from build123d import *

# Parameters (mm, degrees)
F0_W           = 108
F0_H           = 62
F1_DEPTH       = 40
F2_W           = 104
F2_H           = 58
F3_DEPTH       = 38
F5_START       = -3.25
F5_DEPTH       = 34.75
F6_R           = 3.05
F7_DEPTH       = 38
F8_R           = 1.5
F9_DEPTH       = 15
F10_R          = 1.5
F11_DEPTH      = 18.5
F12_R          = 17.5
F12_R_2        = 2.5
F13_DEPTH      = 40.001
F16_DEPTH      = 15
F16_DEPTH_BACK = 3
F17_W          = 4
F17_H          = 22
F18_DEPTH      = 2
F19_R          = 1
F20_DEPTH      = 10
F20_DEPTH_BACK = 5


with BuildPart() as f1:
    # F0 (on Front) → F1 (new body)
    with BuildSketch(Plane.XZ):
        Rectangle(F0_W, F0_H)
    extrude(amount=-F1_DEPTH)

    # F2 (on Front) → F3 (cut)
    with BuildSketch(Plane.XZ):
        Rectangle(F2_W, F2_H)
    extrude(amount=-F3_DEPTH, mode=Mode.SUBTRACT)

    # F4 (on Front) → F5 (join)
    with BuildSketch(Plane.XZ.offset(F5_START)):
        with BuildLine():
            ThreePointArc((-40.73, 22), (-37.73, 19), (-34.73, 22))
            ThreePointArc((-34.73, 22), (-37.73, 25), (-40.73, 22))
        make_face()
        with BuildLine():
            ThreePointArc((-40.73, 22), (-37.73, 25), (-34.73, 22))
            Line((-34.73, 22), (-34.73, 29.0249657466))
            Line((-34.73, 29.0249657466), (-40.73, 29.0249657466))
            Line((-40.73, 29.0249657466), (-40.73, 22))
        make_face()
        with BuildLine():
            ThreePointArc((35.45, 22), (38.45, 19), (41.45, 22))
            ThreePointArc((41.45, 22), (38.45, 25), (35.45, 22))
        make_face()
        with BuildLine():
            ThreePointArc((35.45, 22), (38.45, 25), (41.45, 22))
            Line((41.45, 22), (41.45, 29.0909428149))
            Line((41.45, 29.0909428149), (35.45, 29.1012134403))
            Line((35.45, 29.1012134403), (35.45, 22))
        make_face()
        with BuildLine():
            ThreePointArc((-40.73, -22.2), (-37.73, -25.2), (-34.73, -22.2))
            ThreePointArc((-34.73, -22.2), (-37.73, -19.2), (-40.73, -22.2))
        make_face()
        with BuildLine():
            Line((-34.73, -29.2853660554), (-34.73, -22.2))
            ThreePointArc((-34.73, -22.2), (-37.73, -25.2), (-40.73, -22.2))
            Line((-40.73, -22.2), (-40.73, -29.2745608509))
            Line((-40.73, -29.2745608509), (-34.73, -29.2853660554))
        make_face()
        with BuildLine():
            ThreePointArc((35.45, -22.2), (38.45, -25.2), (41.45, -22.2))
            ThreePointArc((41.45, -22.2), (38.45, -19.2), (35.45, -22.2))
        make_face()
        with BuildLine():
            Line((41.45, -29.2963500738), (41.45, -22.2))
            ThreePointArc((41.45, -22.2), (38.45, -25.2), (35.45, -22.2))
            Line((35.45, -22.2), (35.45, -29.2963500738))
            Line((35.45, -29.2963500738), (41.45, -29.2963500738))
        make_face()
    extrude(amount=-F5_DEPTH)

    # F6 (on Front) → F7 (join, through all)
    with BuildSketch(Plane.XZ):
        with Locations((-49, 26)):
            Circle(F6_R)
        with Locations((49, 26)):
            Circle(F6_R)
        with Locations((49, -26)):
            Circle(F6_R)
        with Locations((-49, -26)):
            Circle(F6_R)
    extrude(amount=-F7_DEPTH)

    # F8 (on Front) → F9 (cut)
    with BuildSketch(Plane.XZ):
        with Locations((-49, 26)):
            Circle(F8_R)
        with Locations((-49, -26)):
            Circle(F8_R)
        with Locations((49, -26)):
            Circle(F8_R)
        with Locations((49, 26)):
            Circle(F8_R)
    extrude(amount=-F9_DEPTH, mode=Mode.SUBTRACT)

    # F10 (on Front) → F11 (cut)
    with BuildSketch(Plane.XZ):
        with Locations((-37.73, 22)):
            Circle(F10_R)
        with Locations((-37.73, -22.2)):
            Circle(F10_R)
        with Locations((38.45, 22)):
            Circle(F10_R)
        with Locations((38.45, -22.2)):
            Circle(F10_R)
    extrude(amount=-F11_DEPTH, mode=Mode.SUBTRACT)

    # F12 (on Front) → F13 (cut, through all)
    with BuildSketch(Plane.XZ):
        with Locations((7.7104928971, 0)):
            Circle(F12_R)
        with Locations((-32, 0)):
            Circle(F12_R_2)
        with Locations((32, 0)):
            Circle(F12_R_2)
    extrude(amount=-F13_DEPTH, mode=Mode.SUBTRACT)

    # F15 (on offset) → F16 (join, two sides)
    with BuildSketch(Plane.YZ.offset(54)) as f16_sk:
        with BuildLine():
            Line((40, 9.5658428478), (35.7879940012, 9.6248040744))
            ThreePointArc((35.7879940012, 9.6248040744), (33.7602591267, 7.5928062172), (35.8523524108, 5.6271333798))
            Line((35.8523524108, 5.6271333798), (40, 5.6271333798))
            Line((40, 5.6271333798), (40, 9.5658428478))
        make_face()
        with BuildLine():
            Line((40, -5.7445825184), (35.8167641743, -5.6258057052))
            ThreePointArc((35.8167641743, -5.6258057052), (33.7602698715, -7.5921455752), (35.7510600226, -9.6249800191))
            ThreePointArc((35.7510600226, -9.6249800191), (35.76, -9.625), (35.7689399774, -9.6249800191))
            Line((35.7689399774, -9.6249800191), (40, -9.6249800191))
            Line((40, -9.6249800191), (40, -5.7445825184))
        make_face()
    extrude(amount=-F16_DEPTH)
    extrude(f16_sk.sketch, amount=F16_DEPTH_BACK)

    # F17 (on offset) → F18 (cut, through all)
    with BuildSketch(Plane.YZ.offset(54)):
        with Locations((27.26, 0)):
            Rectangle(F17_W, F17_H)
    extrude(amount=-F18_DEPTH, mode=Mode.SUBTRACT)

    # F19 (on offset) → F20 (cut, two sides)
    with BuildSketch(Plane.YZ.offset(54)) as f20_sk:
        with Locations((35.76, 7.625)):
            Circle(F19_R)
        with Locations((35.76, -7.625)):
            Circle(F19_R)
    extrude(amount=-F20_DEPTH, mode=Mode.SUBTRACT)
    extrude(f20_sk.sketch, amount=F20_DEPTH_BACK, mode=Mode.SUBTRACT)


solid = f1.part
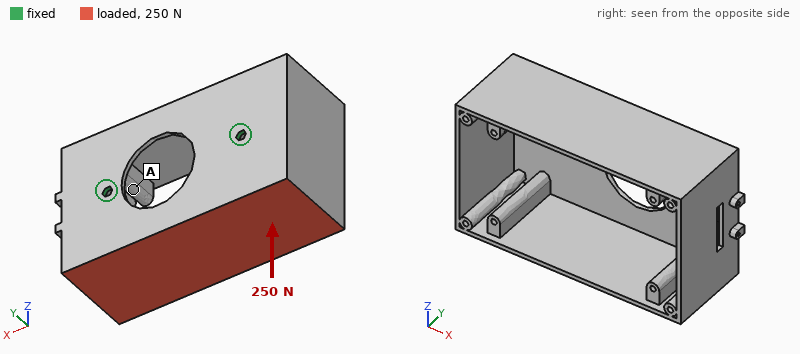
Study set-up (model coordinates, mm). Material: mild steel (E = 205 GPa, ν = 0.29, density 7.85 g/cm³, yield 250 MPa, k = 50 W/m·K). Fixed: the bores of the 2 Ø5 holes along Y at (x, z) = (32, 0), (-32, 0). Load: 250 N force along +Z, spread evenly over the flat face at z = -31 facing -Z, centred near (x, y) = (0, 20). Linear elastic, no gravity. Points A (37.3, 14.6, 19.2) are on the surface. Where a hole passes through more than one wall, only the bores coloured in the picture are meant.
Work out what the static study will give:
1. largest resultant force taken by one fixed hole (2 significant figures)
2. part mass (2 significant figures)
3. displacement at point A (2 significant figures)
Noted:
140 N
380 g
0.063 mm
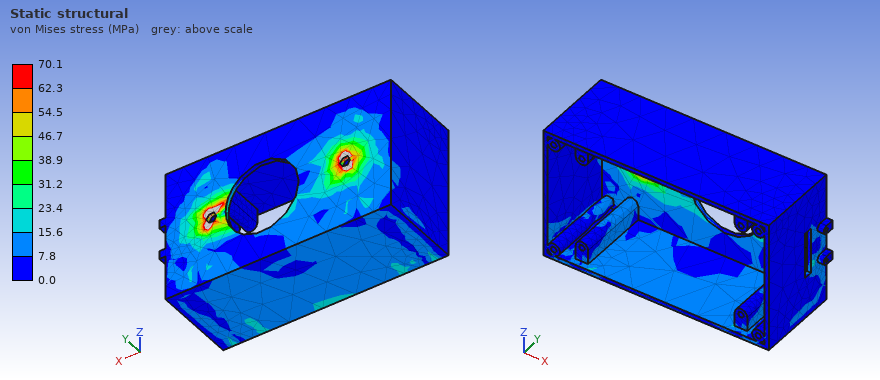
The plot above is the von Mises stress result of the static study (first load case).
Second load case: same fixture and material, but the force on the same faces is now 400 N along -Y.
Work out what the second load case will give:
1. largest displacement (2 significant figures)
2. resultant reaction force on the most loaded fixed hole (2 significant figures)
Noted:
0.28 mm
210 N
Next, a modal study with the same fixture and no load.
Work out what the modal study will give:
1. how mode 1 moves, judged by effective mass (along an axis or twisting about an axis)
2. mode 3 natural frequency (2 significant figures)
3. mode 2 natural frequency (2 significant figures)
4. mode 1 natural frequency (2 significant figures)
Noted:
along Z
1100 Hz
630 Hz
410 Hz
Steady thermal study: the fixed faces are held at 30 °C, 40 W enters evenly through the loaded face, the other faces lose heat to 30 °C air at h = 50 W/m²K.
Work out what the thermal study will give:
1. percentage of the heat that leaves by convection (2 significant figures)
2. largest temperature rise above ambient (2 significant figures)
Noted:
82 %
68 K
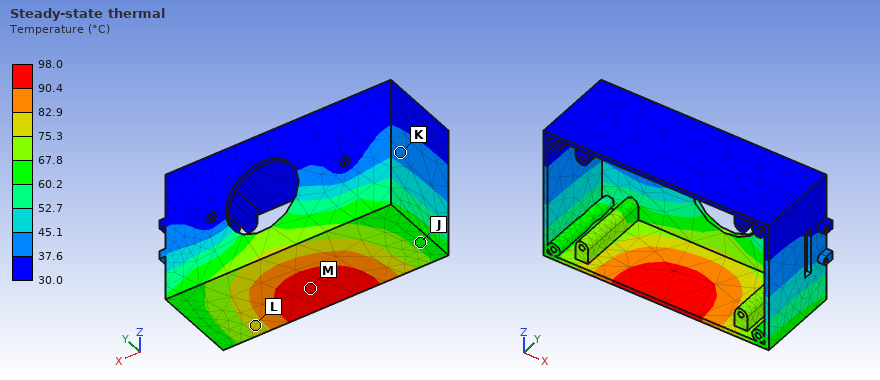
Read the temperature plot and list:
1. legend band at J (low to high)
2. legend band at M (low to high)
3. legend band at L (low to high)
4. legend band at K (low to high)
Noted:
60.2 to 67.8 °C
90.4 to 98.0 °C
75.3 to 82.9 °C
37.6 to 45.1 °C
